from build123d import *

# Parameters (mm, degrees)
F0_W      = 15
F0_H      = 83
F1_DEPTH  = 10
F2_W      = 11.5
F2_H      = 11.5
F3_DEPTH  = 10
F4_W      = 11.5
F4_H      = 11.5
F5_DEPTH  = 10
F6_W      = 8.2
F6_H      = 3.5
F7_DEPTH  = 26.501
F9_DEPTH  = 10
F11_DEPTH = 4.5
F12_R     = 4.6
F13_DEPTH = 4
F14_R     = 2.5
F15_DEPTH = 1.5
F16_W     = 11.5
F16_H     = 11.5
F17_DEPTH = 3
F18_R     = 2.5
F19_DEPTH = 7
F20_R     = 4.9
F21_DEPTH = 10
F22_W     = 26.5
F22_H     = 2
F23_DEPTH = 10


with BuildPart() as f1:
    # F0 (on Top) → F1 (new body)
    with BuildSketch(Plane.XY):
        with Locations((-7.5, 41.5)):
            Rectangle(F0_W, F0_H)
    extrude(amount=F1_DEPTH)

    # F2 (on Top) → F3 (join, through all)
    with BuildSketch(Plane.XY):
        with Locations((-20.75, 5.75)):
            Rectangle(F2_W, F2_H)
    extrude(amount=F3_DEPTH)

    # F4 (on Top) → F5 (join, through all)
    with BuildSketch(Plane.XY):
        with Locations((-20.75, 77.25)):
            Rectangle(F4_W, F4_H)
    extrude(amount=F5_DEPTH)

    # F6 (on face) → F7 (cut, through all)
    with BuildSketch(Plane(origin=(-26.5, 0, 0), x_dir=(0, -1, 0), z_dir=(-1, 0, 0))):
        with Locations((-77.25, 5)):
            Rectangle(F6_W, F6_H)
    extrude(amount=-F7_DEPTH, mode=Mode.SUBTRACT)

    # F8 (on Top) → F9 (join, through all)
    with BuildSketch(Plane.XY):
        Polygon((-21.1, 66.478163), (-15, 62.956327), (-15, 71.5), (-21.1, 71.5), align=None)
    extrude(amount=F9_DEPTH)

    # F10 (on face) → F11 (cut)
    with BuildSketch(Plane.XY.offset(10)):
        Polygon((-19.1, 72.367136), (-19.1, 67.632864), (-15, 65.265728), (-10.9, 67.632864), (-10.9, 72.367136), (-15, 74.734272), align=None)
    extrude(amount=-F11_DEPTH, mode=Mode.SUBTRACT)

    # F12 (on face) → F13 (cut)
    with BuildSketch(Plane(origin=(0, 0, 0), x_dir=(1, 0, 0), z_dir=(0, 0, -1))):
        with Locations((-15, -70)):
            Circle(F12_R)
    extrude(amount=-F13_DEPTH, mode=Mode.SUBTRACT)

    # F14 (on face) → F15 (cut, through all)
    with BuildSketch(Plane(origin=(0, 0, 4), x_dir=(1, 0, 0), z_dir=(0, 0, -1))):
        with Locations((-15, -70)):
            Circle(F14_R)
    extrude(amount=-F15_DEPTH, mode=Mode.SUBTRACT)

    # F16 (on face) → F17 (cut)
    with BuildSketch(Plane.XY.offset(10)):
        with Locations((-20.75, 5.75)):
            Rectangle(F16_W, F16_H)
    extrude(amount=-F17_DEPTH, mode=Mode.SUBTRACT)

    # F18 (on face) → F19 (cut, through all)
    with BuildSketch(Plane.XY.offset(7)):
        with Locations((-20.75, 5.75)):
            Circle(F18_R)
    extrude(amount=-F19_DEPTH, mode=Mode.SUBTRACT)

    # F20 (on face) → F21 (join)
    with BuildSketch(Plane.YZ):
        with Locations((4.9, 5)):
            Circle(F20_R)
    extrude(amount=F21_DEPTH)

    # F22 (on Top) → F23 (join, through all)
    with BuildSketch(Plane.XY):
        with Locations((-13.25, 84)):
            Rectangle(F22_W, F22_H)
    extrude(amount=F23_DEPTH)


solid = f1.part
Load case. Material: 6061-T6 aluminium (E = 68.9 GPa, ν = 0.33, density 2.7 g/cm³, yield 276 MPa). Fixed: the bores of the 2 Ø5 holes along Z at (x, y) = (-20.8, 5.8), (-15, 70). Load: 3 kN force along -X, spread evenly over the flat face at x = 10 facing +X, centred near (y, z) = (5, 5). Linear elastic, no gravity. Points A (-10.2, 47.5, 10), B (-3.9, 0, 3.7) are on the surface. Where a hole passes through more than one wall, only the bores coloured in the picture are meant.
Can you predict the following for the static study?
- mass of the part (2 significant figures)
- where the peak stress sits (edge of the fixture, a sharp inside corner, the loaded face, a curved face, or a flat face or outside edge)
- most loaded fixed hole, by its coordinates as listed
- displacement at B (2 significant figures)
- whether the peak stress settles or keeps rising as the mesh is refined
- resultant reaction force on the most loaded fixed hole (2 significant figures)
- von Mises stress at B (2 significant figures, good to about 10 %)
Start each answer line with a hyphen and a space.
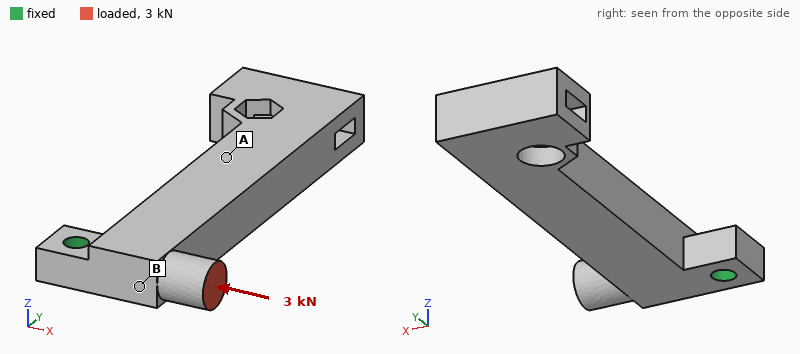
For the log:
- 40 g
- edge of the fixture
- (-20.8, 5.8)
- 17 µm
- keeps rising
- 3.0 kN
- 38 MPa
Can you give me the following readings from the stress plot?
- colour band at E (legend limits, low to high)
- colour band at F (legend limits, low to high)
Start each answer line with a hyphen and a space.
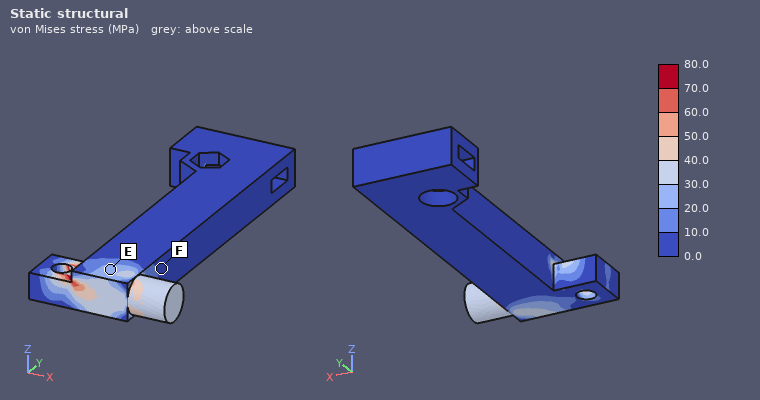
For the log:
- 20.0 to 30.0 MPa
- 0.0 to 10.0 MPa
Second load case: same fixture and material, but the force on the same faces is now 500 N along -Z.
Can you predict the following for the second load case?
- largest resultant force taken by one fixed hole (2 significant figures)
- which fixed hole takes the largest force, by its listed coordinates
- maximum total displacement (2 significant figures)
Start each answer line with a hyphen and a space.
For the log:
- 510 N
- (-20.8, 5.8)
- 0.13 mm
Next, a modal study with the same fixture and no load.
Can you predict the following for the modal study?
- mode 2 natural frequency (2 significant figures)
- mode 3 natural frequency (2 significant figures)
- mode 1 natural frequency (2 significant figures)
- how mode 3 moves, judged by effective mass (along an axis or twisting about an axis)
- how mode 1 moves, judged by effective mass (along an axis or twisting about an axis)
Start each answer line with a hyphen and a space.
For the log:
- 7000 Hz
- 8600 Hz
- 4300 Hz
- twisting about X
- along Z
